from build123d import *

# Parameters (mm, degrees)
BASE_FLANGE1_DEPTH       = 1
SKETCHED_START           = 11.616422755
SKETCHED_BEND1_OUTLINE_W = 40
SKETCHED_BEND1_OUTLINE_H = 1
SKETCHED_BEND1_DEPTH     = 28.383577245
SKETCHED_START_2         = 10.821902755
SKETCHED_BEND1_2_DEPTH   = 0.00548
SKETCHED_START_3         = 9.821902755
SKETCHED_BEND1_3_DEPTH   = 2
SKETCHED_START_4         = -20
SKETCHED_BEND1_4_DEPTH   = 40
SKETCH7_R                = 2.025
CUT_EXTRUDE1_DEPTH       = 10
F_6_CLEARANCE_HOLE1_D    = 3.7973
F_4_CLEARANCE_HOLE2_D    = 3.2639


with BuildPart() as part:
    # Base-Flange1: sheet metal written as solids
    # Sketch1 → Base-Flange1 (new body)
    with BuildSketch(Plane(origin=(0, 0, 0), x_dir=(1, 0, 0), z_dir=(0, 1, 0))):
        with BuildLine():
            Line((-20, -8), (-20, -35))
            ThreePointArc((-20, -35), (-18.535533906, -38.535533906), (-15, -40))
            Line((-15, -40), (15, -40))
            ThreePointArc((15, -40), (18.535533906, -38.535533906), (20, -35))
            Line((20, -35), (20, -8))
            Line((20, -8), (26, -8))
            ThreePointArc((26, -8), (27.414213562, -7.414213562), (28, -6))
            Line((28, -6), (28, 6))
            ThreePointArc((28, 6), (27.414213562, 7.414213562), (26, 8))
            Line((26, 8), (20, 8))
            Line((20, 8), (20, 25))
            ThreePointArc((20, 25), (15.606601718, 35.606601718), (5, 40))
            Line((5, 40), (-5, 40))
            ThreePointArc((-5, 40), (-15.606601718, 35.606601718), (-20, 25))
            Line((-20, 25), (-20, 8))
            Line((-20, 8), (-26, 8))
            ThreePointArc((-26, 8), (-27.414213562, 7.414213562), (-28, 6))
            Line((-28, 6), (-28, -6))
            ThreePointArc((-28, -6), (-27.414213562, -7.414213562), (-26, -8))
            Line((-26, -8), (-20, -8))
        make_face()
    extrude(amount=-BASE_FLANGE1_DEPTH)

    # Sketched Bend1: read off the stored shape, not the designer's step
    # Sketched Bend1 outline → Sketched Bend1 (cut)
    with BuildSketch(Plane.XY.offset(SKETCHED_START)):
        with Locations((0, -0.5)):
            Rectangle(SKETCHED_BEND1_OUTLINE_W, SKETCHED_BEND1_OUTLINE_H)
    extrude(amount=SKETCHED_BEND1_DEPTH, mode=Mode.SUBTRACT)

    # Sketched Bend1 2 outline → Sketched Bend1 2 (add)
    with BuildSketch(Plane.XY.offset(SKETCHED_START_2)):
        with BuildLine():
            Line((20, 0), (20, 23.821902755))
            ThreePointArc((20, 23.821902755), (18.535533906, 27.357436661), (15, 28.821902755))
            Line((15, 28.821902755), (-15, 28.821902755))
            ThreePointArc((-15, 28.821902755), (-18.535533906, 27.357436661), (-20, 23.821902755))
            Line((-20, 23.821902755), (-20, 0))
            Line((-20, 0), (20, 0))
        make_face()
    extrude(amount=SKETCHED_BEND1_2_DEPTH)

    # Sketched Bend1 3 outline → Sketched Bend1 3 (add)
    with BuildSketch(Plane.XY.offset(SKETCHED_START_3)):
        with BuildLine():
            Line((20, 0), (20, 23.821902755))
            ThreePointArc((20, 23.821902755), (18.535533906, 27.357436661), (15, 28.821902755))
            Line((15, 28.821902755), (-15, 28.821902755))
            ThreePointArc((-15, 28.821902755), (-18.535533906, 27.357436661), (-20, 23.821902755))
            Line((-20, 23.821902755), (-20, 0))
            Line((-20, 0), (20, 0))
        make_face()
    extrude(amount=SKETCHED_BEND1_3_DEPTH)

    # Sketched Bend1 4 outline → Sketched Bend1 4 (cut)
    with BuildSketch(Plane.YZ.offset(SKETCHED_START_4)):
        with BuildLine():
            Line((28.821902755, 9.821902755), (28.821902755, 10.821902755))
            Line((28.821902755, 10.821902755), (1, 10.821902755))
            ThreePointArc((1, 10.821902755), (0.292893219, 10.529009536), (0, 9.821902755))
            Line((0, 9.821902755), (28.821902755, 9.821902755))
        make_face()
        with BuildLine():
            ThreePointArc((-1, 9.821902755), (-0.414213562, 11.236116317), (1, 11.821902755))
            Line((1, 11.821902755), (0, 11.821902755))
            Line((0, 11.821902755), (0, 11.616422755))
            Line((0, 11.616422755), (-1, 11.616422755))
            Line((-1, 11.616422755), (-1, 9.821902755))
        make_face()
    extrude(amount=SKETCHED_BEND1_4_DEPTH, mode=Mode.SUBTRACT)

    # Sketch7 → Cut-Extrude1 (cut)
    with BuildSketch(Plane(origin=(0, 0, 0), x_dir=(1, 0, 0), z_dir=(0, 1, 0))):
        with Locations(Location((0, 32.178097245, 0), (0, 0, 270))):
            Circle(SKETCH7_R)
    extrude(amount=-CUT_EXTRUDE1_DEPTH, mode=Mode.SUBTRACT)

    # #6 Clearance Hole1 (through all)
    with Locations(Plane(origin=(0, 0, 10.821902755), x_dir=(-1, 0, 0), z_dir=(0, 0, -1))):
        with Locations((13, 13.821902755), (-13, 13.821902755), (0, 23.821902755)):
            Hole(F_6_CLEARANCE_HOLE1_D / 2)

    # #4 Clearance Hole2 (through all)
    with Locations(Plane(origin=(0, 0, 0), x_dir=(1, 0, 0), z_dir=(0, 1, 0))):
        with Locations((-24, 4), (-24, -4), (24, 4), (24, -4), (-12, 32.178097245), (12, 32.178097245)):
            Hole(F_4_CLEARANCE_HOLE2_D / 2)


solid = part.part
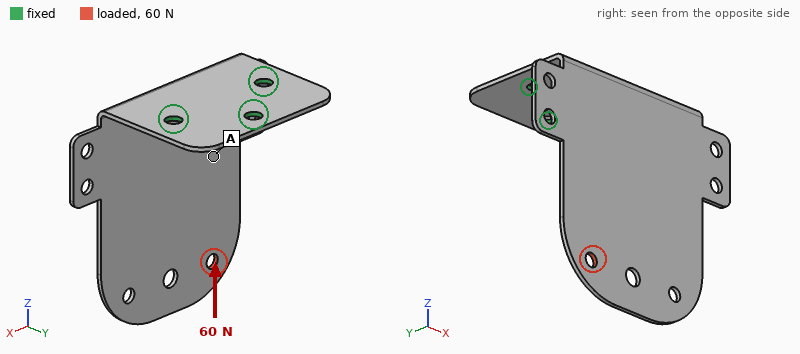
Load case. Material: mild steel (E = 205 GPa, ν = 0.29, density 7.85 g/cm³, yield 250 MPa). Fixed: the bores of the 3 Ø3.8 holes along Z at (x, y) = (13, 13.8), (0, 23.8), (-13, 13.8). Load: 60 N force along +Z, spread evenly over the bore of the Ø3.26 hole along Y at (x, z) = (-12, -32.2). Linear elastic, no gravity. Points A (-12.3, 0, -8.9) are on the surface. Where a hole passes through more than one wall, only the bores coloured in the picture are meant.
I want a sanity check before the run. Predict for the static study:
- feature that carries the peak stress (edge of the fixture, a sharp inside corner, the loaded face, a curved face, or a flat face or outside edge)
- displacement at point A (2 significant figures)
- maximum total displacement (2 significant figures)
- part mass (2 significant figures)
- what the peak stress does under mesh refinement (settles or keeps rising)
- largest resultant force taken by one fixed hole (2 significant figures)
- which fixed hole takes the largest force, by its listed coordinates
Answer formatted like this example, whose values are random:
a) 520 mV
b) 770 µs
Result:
a) edge of the fixture
b) 0.22 mm
c) 0.45 mm
d) 25 g
e) keeps rising
f) 61 N
g) (-13, 13.8)
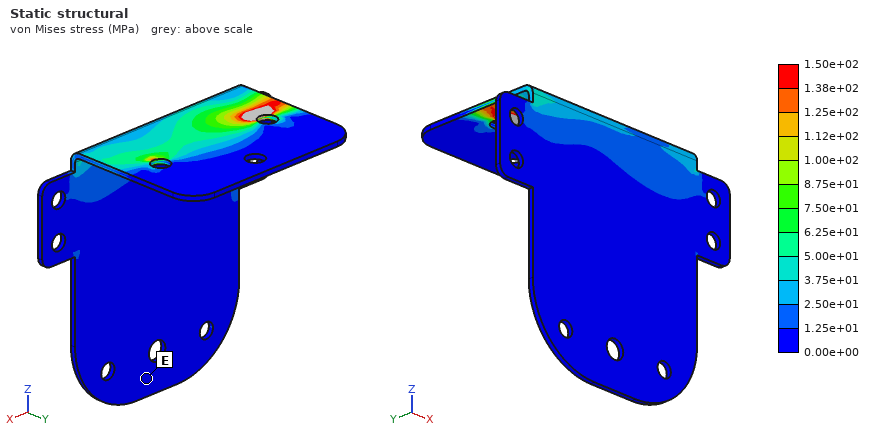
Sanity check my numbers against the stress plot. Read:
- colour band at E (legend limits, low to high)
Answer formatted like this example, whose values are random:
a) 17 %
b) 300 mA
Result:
a) 0.00e+00 to 1.25e+01 MPa
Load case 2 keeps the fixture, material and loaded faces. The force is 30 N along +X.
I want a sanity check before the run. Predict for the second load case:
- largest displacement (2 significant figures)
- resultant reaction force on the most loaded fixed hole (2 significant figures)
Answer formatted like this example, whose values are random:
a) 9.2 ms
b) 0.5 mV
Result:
a) 0.23 mm
b) 51 N
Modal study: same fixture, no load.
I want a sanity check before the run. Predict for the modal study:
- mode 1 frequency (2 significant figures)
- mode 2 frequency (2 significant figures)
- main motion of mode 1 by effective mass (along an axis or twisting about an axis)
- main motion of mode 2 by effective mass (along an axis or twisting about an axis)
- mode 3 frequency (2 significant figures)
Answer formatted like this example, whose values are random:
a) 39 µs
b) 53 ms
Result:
a) 250 Hz
b) 660 Hz
c) along Y
d) along X
e) 1100 Hz
